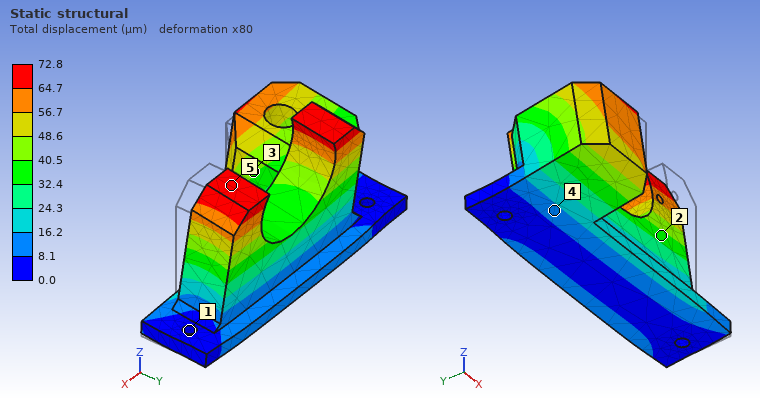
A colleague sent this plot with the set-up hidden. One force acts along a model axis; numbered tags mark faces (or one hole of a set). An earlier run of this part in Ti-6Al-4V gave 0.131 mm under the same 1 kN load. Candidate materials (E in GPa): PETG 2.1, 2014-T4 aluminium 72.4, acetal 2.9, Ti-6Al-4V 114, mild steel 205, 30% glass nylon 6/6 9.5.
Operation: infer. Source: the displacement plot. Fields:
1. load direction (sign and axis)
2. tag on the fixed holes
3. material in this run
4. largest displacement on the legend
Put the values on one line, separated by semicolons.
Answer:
+Y; 1; mild steel; 72.8 µm
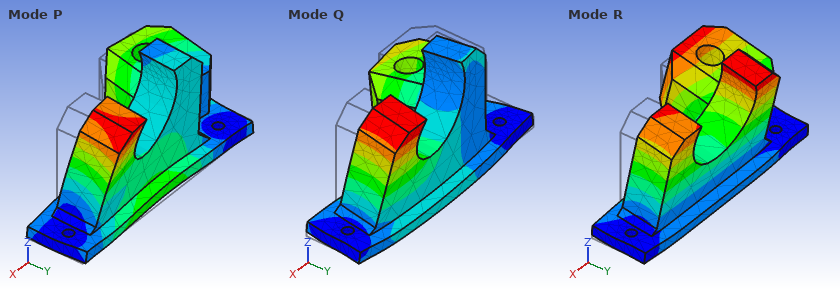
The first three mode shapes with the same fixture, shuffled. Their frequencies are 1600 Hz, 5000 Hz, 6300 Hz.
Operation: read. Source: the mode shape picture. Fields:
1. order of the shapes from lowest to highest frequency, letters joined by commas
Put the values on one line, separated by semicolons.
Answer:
R, Q, P
